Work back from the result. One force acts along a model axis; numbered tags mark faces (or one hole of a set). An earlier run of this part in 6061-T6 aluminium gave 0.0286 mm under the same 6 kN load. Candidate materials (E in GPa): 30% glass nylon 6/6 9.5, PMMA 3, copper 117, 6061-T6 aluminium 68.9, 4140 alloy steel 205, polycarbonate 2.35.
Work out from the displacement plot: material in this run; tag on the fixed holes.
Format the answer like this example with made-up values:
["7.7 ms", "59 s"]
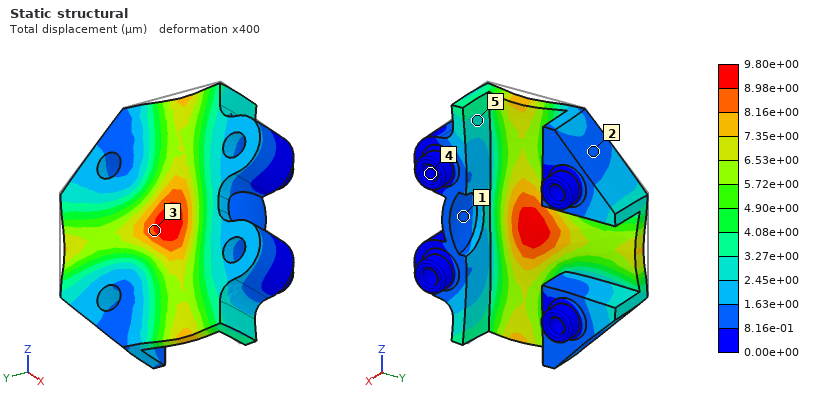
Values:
["4140 alloy steel", "4"]
